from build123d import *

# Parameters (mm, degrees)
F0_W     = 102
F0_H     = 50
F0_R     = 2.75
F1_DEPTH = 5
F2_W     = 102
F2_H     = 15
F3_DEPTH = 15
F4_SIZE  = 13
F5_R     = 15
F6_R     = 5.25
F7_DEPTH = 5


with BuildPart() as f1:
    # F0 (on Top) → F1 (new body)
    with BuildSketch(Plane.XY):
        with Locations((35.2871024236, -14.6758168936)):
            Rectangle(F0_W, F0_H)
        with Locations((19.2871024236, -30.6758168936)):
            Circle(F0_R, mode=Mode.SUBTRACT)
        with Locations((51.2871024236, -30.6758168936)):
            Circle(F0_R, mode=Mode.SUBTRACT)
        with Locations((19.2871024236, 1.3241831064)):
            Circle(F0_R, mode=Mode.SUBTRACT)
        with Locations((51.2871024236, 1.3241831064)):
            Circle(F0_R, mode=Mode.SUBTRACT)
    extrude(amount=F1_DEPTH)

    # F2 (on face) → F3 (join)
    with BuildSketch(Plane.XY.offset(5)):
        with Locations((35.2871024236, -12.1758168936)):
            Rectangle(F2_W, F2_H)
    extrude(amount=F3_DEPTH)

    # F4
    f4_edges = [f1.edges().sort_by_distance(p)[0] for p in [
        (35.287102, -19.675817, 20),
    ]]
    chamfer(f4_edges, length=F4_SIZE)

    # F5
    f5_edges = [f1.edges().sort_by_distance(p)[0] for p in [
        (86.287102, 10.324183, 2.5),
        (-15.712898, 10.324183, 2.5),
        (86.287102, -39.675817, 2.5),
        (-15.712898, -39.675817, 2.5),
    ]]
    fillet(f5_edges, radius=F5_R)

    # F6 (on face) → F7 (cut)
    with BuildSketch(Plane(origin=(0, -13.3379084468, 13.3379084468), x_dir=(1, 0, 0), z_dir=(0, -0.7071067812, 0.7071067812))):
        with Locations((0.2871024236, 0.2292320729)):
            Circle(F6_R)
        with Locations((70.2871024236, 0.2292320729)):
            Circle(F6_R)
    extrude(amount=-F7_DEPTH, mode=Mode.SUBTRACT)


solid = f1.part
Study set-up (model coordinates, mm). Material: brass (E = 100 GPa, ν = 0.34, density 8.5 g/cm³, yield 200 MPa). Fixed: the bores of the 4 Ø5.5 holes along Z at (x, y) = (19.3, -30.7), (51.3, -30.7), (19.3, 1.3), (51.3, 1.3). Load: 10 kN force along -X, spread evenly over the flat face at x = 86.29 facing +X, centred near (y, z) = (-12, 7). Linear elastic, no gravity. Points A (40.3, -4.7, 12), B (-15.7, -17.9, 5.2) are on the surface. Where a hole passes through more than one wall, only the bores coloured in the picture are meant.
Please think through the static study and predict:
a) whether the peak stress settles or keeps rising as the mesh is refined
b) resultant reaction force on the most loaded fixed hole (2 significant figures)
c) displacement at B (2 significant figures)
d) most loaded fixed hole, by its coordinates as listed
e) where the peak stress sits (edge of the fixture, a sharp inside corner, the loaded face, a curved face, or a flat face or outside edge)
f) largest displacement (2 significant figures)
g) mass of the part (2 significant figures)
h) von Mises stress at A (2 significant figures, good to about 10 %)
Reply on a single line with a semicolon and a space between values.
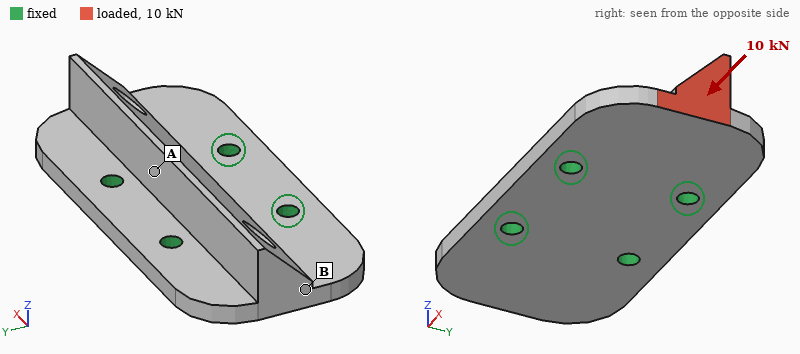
keeps rising; 4.0 kN; 15 µm; (51.3, 1.3); edge of the fixture; 62 µm; 320 g; 27 MPa
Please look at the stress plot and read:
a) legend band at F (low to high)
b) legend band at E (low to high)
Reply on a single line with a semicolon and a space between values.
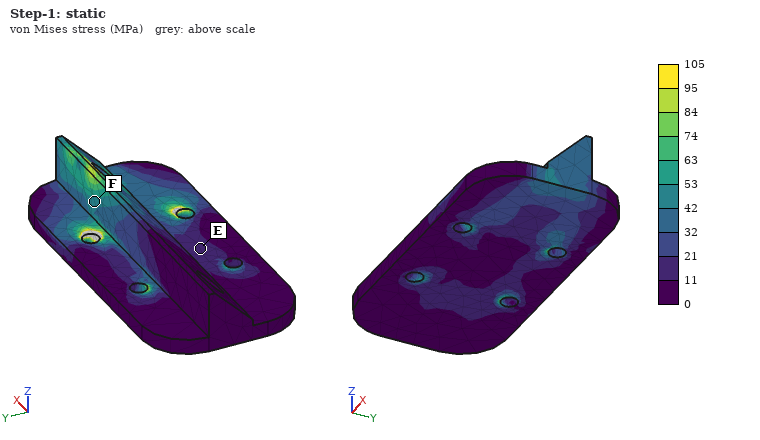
42 to 53 MPa; 11 to 21 MPa
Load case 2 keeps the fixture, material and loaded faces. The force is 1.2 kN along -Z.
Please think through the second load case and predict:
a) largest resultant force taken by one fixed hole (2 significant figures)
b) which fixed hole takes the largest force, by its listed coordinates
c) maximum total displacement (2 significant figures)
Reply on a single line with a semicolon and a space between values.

1.7 kN; (51.3, 1.3); 68 µm
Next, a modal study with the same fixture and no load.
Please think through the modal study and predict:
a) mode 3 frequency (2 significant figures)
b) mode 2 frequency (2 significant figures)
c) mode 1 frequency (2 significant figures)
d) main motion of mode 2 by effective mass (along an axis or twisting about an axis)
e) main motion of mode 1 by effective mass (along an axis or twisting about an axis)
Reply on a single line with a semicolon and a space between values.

6300 Hz; 4200 Hz; 3500 Hz; along Z; twisting about Y
